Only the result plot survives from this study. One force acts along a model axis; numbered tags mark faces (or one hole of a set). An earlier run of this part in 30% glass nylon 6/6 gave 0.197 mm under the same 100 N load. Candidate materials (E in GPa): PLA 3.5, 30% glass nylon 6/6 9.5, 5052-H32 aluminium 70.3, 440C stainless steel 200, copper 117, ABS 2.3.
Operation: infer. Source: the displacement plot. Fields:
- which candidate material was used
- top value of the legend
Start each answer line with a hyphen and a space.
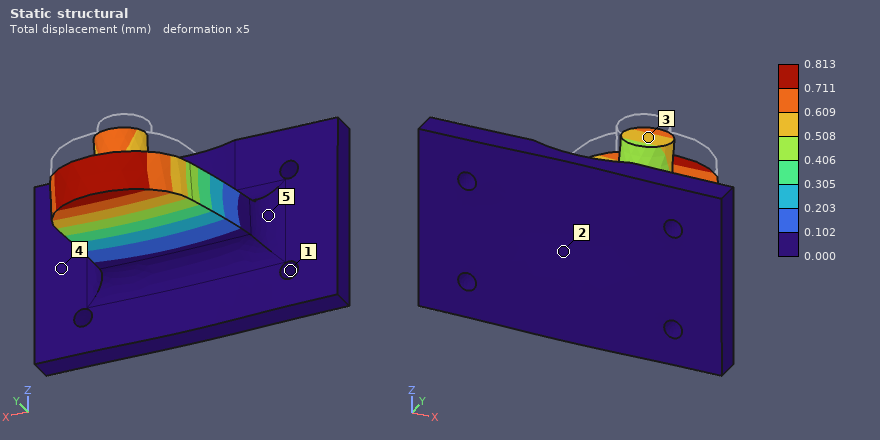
- ABS
- 0.813 mm
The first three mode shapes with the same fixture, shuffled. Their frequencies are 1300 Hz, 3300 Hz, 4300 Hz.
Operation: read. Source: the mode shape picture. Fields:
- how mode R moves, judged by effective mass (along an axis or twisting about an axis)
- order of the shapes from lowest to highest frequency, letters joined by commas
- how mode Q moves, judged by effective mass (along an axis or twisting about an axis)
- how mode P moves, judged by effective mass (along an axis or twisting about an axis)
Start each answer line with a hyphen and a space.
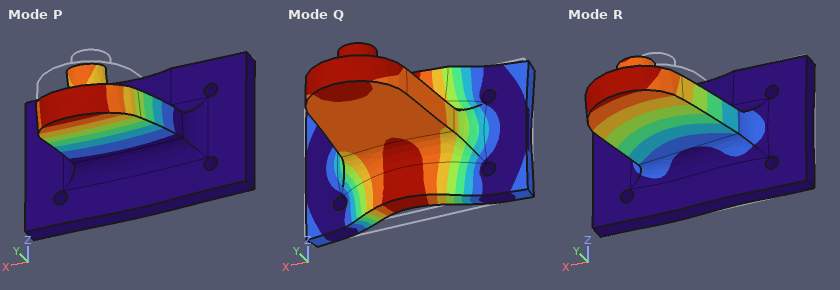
- along X
- P, R, Q
- along Y
- along Z
